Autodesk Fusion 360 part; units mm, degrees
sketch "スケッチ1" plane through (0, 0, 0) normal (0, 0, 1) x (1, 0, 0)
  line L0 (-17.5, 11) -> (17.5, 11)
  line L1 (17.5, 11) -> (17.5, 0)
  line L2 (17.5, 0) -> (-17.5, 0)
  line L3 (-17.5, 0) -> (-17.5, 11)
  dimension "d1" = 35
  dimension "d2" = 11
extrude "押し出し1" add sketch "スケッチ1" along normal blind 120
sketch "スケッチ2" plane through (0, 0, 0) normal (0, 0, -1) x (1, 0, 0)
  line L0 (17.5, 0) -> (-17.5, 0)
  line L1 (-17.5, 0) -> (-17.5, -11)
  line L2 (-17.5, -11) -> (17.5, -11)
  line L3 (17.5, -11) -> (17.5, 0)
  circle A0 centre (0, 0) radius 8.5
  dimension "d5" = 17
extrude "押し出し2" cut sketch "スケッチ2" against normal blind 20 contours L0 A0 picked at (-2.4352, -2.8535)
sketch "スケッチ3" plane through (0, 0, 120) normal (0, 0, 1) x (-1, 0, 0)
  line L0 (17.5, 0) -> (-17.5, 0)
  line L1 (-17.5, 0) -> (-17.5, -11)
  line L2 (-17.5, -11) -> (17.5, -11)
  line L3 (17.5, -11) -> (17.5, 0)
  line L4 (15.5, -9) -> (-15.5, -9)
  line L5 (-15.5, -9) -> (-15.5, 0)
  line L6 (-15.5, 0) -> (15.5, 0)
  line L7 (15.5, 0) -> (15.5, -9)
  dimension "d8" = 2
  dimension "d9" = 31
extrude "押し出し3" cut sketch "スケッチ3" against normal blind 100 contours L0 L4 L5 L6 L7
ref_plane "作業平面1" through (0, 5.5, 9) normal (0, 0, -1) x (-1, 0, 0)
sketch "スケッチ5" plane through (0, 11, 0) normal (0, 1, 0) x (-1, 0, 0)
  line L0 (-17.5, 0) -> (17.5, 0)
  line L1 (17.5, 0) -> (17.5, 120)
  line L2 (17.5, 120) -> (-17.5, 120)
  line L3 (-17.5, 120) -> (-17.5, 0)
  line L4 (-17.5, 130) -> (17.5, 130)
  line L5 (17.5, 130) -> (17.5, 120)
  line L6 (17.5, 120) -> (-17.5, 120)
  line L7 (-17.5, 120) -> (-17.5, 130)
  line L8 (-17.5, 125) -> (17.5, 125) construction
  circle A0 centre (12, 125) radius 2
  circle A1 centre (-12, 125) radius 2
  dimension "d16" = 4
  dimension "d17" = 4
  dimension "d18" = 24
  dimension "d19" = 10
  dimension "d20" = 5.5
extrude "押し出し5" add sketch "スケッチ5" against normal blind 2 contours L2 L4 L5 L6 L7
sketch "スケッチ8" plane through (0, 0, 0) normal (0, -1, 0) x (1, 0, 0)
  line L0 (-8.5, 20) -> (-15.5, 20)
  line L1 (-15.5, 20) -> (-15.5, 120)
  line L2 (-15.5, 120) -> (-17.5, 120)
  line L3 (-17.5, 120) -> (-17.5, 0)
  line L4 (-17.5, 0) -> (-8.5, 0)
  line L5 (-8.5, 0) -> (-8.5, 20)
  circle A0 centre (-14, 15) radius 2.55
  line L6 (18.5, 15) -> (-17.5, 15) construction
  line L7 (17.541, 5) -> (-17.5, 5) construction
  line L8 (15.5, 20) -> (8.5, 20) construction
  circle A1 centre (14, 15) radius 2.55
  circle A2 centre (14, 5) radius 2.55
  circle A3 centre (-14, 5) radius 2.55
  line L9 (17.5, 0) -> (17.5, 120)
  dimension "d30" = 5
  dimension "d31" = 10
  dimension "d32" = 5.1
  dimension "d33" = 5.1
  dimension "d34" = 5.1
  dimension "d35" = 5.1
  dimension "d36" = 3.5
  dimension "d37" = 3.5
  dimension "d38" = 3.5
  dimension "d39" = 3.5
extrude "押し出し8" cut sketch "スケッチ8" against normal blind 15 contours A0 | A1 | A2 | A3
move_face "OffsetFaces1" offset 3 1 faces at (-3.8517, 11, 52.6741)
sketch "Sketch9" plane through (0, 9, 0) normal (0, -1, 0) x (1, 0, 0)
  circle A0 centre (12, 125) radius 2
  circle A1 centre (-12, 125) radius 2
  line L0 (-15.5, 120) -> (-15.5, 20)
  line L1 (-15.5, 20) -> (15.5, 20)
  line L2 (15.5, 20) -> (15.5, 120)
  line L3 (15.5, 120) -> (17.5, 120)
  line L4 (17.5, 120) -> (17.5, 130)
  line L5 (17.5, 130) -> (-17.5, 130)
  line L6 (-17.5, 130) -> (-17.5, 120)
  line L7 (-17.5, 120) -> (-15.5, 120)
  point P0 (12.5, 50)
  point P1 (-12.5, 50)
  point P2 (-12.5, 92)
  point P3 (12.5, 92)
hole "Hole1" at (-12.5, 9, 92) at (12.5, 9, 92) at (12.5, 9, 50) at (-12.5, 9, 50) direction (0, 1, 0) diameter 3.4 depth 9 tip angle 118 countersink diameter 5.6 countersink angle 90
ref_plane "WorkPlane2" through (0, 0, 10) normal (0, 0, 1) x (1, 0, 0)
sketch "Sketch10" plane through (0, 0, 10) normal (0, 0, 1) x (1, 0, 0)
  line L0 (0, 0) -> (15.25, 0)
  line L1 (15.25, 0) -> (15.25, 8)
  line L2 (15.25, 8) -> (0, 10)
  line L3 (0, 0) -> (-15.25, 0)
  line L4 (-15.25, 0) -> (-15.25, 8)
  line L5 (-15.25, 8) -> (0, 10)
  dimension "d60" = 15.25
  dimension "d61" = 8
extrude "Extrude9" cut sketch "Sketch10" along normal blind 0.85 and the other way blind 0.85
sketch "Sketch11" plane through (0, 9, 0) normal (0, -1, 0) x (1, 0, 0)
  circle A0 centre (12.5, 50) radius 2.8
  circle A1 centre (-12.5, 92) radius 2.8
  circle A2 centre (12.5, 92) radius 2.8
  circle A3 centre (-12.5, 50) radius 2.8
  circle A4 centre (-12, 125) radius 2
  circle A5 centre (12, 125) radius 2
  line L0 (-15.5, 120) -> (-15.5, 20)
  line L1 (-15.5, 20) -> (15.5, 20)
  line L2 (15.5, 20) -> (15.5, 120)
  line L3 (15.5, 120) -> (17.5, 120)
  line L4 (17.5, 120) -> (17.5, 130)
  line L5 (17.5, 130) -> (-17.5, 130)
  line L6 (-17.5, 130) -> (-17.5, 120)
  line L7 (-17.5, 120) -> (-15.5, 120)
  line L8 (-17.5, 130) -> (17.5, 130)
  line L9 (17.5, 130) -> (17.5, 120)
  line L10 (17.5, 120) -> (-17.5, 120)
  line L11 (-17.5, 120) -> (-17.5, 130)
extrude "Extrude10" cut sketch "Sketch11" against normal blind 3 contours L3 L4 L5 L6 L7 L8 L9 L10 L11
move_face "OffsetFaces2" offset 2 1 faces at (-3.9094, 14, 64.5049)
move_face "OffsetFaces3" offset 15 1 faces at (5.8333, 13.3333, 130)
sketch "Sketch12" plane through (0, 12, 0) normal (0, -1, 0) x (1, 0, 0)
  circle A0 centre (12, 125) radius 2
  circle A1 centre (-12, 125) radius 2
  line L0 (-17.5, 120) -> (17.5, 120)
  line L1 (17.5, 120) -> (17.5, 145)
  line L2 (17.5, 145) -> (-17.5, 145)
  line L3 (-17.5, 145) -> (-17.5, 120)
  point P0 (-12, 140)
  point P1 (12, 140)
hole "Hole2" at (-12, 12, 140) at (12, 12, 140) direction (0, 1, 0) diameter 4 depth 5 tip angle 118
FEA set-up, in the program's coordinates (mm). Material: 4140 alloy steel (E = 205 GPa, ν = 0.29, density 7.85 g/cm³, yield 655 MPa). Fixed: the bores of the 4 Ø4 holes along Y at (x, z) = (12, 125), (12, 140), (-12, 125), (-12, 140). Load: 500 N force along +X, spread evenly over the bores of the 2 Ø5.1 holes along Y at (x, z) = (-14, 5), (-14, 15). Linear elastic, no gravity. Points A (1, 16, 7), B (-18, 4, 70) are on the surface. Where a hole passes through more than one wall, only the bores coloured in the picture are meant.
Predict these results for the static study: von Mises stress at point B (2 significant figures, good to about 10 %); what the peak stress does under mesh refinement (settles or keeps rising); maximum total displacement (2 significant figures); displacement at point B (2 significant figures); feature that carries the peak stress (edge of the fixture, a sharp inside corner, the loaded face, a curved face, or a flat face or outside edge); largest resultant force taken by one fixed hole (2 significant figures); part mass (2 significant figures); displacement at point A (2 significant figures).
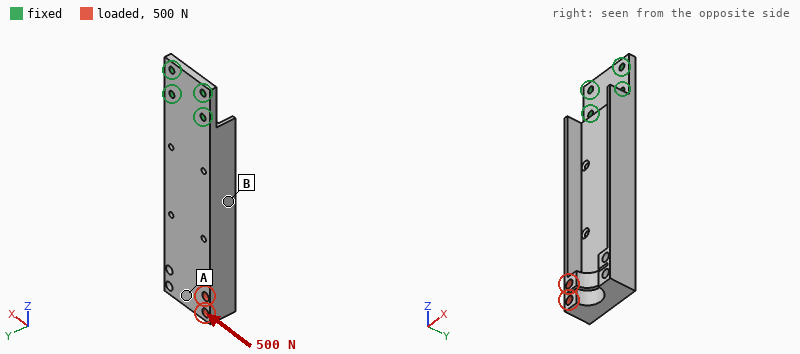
13 MPa
keeps rising
73 µm
21 µm
edge of the fixture
2.1 kN
300 g
58 µm
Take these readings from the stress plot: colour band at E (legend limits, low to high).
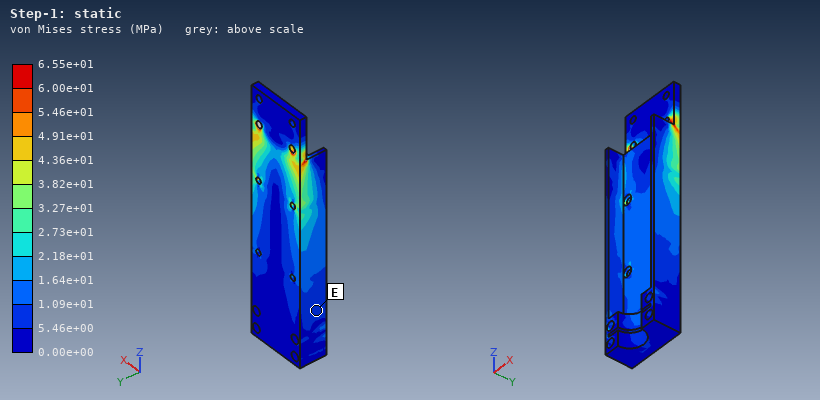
5.46e+00 to 1.09e+01 MPa
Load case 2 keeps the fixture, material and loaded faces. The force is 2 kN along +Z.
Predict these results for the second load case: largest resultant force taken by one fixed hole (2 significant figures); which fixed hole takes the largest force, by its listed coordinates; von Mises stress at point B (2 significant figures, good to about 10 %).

1.9 kN
(-12, 125)
36 MPa
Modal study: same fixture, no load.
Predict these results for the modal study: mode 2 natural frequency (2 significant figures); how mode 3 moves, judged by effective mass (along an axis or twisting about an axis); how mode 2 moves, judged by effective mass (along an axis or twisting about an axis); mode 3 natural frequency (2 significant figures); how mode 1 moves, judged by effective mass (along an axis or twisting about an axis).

1400 Hz
twisting about Z
along X
1900 Hz
along Y
